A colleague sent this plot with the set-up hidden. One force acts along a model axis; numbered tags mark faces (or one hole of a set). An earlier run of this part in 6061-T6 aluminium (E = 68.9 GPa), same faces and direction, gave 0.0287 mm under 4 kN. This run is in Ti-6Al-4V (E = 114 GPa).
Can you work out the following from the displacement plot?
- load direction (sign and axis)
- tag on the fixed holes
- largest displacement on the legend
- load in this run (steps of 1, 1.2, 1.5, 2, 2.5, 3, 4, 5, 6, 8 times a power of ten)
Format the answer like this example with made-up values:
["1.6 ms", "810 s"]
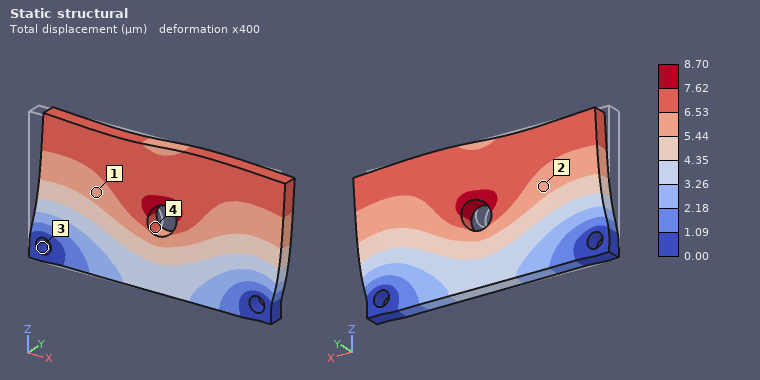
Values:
["+X", "3", "8.70 µm", "2 kN"]
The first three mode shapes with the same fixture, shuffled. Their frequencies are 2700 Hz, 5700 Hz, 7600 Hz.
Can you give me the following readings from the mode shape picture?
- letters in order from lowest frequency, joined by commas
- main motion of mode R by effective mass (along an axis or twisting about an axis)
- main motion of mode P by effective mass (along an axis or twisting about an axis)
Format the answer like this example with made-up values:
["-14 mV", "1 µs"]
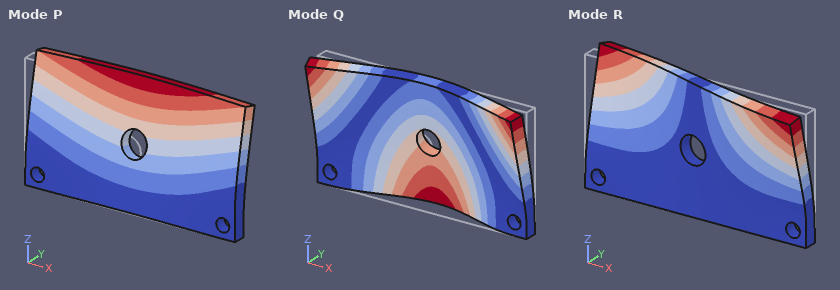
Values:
["P, R, Q", "twisting about Z", "along Y"]
